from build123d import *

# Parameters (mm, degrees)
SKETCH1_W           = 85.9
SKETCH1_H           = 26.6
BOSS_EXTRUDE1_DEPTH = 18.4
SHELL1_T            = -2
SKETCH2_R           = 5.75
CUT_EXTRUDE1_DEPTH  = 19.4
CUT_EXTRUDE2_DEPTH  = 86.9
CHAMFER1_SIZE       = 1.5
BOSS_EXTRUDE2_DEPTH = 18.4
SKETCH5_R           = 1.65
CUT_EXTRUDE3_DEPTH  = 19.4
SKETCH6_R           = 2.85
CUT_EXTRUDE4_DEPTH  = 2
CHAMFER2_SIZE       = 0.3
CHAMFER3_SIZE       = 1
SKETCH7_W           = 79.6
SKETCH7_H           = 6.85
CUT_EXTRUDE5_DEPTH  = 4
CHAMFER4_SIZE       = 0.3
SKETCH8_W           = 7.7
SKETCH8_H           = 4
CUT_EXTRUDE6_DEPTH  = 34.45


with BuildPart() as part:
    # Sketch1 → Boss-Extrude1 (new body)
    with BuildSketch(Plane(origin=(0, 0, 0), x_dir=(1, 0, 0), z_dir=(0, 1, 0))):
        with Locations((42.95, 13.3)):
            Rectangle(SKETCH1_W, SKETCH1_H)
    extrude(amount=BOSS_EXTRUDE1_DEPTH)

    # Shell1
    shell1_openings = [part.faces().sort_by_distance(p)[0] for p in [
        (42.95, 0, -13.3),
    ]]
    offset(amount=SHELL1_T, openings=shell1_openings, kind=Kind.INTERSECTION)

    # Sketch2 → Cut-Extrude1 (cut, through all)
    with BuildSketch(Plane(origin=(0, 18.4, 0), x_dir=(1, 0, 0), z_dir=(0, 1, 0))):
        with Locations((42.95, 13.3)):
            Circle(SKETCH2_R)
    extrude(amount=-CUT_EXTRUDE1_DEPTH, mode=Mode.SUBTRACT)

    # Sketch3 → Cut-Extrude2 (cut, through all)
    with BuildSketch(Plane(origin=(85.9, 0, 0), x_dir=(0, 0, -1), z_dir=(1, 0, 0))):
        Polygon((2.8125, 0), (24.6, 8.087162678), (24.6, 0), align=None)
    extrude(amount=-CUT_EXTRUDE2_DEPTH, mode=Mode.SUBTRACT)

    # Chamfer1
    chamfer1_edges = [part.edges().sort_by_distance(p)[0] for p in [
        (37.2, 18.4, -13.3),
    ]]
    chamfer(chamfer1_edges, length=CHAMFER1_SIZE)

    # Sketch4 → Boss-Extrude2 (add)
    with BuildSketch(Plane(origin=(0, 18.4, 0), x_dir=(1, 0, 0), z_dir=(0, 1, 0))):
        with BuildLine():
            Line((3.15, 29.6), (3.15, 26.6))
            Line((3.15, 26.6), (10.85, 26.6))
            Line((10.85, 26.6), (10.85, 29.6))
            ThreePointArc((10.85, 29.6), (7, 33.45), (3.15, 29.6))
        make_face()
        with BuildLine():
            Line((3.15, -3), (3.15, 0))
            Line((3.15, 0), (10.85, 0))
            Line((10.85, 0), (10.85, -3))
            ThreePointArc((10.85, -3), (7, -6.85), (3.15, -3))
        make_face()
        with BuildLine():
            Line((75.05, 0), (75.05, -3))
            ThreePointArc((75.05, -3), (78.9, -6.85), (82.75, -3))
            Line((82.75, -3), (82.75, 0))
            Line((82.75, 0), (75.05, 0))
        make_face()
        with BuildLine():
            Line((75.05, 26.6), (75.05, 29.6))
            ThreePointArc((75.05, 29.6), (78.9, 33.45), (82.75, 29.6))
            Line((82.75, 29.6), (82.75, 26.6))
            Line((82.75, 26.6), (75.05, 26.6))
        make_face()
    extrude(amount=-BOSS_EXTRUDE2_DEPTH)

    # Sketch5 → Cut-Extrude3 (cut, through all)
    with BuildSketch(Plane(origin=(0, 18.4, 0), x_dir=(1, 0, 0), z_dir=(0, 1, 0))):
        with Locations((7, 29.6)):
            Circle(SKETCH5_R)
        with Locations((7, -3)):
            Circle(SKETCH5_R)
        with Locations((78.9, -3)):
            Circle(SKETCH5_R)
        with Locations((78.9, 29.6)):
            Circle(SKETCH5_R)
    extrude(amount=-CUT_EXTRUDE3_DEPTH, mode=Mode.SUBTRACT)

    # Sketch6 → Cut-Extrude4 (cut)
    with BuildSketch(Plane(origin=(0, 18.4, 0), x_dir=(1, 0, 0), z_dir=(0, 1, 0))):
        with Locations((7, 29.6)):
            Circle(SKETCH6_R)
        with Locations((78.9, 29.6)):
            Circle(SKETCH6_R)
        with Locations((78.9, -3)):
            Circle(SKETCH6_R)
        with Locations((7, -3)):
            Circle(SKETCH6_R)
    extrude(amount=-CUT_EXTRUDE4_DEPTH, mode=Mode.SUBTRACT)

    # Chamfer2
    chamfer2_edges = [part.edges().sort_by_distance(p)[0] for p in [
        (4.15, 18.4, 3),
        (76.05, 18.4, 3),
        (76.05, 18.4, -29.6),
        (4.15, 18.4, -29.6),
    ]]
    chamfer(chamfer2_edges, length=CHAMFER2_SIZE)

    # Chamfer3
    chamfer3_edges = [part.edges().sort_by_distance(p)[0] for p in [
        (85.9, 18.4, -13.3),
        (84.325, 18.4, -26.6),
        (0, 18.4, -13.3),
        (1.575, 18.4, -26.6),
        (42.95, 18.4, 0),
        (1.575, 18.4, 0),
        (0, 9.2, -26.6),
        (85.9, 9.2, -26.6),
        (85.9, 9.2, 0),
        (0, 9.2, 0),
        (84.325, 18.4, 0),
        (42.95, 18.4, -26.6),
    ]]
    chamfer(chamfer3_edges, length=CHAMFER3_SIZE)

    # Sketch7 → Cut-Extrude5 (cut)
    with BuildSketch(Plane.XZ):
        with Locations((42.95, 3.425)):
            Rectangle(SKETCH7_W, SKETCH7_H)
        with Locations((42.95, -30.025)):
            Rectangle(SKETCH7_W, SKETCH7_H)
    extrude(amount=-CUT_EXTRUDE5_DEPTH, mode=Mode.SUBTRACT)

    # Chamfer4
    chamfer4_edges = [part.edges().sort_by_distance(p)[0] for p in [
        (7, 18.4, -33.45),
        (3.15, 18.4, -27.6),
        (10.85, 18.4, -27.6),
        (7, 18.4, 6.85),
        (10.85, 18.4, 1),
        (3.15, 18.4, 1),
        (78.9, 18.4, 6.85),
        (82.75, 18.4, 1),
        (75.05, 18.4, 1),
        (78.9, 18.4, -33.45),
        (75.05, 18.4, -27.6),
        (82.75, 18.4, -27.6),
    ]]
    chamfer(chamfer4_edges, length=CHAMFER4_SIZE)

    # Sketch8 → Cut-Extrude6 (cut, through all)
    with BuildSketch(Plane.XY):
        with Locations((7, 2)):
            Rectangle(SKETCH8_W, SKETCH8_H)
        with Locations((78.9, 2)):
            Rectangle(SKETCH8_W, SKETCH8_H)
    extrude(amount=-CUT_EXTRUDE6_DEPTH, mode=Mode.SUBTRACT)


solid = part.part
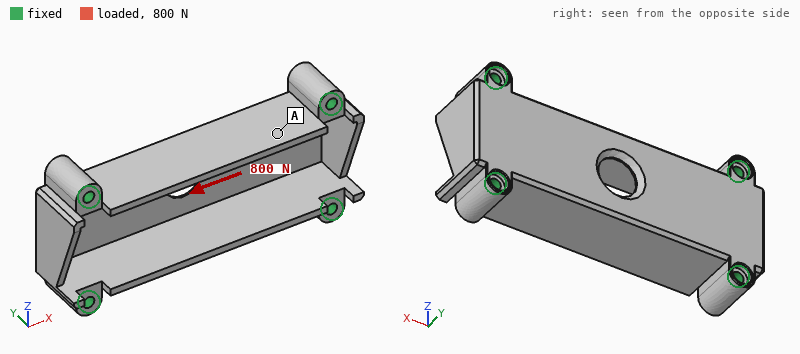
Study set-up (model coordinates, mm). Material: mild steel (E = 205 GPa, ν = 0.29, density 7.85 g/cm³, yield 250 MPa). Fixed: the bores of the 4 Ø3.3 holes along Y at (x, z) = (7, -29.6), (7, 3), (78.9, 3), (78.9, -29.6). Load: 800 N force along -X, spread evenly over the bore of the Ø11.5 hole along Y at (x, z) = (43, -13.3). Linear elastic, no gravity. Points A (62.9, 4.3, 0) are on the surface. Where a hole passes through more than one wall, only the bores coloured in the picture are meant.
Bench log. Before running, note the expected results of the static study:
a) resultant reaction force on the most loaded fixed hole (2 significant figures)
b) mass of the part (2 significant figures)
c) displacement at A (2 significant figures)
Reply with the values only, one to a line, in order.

200 N
100 g
0.56 µm
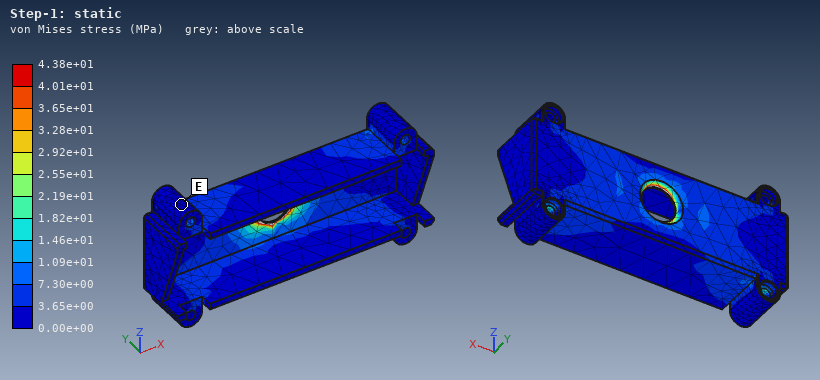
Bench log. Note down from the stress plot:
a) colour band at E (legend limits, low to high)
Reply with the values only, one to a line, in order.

0.00e+00 to 3.65e+00 MPa
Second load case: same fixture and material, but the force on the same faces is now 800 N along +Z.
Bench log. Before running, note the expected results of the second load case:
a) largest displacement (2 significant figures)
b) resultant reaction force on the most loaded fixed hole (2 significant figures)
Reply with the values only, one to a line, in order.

6.3 µm
320 N
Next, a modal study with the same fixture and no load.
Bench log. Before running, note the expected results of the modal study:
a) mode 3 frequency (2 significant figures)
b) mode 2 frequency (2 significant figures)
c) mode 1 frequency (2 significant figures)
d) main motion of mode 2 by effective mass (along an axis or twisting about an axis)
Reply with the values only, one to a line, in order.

8600 Hz
5100 Hz
4400 Hz
along Z
